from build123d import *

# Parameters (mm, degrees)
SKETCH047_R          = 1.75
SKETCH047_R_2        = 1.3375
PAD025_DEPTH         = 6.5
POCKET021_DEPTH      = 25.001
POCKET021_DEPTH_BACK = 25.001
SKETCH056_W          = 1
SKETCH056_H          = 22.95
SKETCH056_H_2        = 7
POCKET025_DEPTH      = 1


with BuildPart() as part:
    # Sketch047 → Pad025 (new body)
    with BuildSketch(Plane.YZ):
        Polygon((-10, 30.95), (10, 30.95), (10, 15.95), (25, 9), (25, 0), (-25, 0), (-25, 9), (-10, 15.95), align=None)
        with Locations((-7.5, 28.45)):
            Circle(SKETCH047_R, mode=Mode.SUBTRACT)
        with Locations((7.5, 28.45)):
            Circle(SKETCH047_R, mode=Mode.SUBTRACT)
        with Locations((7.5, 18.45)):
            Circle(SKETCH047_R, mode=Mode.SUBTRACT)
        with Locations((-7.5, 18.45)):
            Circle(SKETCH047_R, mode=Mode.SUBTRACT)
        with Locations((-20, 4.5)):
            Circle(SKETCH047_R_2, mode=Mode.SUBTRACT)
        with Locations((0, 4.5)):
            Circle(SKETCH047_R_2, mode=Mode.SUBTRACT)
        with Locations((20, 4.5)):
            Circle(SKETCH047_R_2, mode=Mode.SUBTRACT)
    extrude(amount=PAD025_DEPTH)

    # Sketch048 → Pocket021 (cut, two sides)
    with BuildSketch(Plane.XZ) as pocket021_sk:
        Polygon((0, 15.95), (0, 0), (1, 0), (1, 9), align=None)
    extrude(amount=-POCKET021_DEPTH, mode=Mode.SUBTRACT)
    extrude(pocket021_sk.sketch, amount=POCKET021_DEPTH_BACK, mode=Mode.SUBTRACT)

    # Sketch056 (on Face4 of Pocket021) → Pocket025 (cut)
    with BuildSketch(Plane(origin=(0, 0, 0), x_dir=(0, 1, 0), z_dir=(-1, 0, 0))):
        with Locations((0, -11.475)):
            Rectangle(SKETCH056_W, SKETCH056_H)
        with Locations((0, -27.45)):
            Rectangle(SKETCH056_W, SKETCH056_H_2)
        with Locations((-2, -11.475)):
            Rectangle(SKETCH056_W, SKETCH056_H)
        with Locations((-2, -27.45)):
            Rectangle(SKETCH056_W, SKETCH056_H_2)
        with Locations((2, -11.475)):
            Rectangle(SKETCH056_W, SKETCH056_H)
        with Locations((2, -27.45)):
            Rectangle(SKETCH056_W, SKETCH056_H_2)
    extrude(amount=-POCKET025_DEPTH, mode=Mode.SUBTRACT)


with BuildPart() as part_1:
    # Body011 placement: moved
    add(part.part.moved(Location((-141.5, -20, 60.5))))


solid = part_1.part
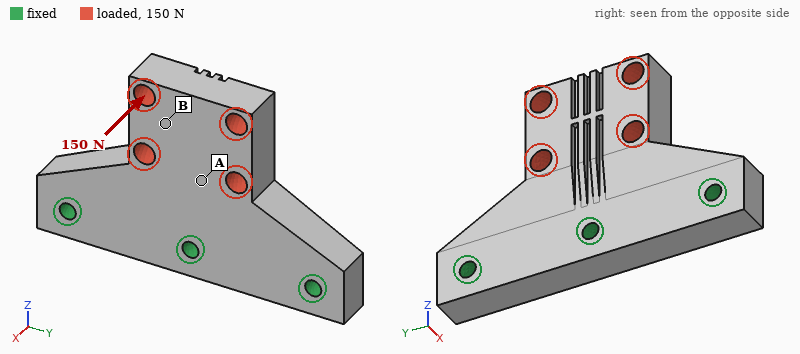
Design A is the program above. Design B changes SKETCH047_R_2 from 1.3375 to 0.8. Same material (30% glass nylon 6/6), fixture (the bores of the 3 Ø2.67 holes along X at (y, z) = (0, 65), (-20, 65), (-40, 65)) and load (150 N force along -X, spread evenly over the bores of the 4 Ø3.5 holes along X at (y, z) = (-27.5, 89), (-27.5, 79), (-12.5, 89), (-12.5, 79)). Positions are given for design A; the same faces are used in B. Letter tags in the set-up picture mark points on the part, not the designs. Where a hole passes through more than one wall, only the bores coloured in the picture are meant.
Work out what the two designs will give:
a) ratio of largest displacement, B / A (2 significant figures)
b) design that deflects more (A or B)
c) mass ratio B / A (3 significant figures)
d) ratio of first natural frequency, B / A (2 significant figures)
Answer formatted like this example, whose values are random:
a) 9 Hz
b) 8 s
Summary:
a) 1.2
b) B
c) 1.01
d) 0.92
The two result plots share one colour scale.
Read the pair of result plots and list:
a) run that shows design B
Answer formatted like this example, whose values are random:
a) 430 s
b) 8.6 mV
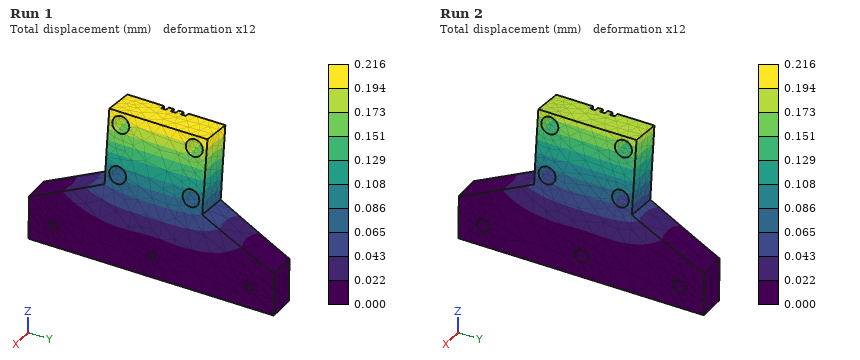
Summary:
a) Run 1
